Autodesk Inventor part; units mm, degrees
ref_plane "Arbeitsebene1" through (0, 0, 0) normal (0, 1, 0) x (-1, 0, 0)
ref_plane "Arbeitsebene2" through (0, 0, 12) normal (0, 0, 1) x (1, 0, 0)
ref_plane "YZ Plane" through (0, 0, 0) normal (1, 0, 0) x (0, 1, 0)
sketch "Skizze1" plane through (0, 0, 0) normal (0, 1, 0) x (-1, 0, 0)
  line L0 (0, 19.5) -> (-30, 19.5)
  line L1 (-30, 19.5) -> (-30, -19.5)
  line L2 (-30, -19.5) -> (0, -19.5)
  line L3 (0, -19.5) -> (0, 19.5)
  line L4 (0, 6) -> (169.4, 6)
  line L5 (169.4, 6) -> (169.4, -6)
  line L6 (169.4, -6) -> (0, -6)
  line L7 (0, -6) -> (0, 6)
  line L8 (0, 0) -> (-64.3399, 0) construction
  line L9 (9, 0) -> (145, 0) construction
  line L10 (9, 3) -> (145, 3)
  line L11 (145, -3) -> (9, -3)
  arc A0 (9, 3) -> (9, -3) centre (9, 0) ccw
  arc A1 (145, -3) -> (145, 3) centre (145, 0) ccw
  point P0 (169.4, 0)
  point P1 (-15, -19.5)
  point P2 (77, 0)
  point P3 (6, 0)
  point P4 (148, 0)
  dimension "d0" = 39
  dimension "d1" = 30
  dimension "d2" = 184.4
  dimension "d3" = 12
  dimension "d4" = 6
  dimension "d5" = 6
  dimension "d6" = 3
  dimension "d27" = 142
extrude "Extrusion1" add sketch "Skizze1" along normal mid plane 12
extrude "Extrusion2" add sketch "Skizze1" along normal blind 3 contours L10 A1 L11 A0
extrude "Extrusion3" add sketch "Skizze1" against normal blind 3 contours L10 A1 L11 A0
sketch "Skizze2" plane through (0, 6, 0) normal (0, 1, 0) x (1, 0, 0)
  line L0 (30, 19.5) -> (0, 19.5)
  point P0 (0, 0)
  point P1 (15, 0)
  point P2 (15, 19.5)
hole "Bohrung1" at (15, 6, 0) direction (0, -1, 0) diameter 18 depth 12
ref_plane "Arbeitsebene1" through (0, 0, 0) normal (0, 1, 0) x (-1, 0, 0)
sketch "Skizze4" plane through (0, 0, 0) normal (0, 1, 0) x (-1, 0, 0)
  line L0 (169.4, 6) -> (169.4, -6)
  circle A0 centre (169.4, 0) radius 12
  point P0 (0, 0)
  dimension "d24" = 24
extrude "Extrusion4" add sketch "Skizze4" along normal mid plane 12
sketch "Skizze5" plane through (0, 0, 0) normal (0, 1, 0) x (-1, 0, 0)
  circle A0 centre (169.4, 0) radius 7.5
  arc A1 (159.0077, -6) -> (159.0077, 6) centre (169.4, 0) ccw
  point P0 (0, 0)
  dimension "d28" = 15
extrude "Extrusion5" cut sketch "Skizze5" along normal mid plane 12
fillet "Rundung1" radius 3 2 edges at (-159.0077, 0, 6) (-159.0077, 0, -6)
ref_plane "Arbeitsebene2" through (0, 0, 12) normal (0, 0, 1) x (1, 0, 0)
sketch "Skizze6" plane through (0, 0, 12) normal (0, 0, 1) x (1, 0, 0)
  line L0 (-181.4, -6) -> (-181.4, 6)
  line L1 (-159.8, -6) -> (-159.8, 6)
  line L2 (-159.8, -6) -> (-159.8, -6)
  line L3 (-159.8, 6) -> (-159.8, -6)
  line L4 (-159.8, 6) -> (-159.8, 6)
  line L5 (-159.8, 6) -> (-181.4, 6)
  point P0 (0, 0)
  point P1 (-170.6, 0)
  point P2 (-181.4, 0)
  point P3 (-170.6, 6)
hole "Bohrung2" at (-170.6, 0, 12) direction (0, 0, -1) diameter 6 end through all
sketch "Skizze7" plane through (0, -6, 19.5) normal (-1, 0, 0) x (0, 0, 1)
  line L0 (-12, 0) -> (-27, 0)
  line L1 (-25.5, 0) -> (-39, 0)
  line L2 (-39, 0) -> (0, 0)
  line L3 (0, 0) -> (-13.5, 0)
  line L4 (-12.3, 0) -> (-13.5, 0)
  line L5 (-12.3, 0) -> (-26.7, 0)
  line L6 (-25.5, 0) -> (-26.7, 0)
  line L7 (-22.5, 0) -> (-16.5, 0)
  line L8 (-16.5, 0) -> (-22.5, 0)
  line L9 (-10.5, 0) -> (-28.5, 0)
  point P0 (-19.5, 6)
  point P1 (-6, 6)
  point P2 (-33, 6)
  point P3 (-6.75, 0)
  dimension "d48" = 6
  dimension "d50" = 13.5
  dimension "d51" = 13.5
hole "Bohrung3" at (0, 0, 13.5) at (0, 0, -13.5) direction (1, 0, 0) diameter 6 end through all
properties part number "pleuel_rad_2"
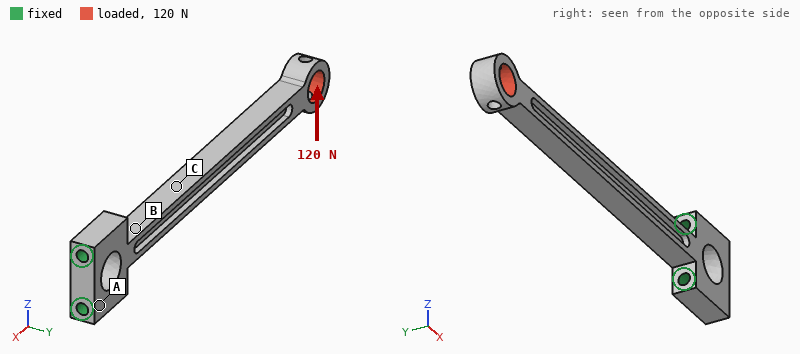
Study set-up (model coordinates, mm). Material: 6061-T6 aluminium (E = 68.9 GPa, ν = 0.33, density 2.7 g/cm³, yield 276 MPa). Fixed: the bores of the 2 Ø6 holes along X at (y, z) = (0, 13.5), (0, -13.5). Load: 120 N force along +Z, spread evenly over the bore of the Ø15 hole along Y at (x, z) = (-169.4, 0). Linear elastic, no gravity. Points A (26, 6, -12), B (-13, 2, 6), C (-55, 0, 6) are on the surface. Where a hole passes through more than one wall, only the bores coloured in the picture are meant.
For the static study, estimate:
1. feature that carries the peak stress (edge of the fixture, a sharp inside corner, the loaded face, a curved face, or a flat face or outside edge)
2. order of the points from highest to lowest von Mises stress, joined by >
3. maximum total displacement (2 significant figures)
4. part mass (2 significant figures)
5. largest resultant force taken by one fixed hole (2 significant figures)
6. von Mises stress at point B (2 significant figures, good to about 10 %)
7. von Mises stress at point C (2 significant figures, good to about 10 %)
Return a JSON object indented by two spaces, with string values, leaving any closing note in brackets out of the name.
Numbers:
{
  "feature that carries the peak stress": "a flat face or outside edge",
  "order of the points from highest to lowest von Mises stress, joined by >": "B > C > A",
  "maximum total displacement": "2.1 mm",
  "part mass": "81 g",
  "largest resultant force taken by one fixed hole": "1.3 kN",
  "von Mises stress at point B": "69 MPa",
  "von Mises stress at point C": "51 MPa"
}
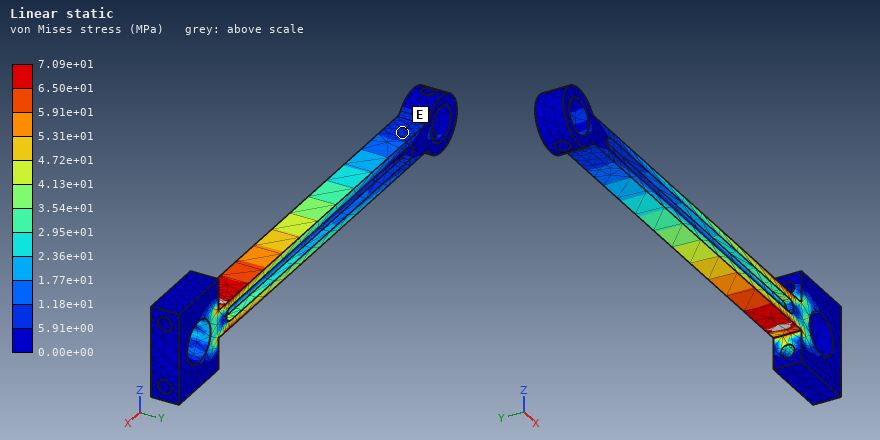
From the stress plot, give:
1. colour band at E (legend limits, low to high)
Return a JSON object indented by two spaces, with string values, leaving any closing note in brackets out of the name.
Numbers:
{
  "colour band at E": "5.91e+00 to 1.18e+01 MPa"
}
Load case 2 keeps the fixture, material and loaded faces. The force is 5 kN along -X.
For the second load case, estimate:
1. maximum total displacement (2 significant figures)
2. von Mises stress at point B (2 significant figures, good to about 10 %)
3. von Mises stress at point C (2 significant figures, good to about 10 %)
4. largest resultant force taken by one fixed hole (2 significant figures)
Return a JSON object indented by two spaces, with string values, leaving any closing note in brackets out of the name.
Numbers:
{
  "maximum total displacement": "0.16 mm",
  "von Mises stress at point B": "45 MPa",
  "von Mises stress at point C": "46 MPa",
  "largest resultant force taken by one fixed hole": "2.8 kN"
}
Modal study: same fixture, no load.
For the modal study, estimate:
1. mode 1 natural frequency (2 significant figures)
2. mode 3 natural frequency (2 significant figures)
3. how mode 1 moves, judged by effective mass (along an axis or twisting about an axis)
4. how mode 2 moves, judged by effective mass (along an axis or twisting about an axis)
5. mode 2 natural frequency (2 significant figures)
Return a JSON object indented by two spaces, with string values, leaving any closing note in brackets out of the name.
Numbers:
{
  "mode 1 natural frequency": "230 Hz",
  "mode 3 natural frequency": "1500 Hz",
  "how mode 1 moves, judged by effective mass": "along Y",
  "how mode 2 moves, judged by effective mass": "along Z",
  "mode 2 natural frequency": "300 Hz"
}
